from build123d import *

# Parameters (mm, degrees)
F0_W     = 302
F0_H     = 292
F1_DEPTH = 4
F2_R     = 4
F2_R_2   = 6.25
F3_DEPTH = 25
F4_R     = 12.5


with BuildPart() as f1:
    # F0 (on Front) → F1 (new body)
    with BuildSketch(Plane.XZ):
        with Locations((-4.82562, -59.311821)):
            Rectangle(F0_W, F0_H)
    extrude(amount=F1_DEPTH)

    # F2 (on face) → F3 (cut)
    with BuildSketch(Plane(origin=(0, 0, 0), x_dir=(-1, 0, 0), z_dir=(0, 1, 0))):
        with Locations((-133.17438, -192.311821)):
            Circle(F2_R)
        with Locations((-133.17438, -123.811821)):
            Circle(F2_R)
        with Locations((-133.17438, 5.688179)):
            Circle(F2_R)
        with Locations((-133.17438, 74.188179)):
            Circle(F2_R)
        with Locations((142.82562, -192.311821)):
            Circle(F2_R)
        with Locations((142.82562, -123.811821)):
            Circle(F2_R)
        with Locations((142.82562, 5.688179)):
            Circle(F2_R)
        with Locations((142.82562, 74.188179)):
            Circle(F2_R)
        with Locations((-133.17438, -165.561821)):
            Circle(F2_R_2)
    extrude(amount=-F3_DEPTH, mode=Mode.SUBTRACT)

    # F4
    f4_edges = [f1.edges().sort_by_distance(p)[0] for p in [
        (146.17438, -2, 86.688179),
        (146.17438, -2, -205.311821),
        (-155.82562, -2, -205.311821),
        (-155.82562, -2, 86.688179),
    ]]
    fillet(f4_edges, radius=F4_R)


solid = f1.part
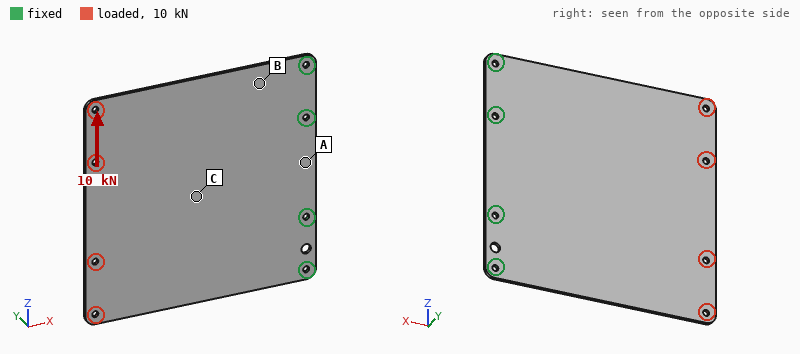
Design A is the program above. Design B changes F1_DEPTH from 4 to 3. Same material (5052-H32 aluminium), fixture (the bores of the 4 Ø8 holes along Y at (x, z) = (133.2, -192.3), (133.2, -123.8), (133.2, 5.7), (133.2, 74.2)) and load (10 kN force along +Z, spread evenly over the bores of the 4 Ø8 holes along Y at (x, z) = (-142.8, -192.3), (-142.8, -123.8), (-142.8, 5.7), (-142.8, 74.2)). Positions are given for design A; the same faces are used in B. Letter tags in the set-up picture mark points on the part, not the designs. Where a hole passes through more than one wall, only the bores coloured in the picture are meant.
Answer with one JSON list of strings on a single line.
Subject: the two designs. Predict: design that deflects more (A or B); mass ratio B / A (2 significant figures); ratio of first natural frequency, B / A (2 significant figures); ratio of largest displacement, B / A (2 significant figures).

["B", "0.75", "0.75", "1.3"]
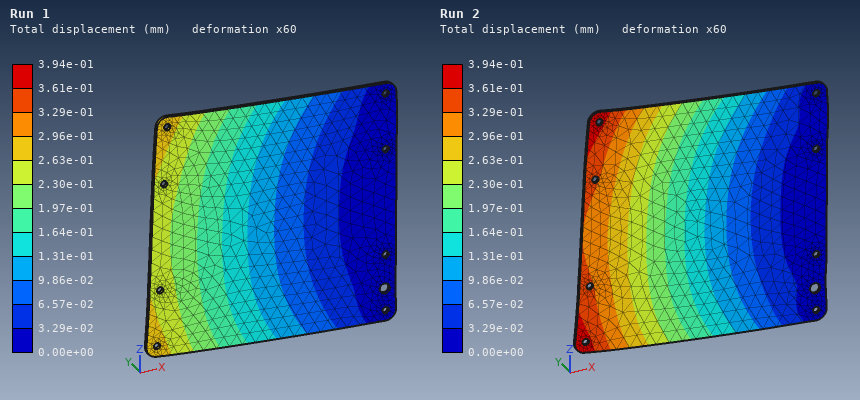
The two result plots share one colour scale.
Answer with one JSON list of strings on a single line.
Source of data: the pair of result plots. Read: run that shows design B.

["Run 2"]
